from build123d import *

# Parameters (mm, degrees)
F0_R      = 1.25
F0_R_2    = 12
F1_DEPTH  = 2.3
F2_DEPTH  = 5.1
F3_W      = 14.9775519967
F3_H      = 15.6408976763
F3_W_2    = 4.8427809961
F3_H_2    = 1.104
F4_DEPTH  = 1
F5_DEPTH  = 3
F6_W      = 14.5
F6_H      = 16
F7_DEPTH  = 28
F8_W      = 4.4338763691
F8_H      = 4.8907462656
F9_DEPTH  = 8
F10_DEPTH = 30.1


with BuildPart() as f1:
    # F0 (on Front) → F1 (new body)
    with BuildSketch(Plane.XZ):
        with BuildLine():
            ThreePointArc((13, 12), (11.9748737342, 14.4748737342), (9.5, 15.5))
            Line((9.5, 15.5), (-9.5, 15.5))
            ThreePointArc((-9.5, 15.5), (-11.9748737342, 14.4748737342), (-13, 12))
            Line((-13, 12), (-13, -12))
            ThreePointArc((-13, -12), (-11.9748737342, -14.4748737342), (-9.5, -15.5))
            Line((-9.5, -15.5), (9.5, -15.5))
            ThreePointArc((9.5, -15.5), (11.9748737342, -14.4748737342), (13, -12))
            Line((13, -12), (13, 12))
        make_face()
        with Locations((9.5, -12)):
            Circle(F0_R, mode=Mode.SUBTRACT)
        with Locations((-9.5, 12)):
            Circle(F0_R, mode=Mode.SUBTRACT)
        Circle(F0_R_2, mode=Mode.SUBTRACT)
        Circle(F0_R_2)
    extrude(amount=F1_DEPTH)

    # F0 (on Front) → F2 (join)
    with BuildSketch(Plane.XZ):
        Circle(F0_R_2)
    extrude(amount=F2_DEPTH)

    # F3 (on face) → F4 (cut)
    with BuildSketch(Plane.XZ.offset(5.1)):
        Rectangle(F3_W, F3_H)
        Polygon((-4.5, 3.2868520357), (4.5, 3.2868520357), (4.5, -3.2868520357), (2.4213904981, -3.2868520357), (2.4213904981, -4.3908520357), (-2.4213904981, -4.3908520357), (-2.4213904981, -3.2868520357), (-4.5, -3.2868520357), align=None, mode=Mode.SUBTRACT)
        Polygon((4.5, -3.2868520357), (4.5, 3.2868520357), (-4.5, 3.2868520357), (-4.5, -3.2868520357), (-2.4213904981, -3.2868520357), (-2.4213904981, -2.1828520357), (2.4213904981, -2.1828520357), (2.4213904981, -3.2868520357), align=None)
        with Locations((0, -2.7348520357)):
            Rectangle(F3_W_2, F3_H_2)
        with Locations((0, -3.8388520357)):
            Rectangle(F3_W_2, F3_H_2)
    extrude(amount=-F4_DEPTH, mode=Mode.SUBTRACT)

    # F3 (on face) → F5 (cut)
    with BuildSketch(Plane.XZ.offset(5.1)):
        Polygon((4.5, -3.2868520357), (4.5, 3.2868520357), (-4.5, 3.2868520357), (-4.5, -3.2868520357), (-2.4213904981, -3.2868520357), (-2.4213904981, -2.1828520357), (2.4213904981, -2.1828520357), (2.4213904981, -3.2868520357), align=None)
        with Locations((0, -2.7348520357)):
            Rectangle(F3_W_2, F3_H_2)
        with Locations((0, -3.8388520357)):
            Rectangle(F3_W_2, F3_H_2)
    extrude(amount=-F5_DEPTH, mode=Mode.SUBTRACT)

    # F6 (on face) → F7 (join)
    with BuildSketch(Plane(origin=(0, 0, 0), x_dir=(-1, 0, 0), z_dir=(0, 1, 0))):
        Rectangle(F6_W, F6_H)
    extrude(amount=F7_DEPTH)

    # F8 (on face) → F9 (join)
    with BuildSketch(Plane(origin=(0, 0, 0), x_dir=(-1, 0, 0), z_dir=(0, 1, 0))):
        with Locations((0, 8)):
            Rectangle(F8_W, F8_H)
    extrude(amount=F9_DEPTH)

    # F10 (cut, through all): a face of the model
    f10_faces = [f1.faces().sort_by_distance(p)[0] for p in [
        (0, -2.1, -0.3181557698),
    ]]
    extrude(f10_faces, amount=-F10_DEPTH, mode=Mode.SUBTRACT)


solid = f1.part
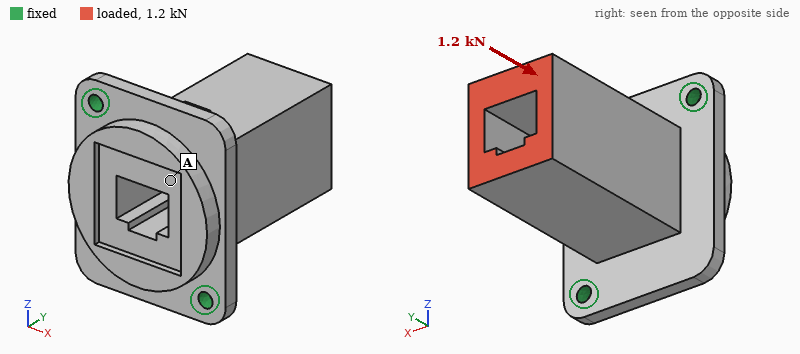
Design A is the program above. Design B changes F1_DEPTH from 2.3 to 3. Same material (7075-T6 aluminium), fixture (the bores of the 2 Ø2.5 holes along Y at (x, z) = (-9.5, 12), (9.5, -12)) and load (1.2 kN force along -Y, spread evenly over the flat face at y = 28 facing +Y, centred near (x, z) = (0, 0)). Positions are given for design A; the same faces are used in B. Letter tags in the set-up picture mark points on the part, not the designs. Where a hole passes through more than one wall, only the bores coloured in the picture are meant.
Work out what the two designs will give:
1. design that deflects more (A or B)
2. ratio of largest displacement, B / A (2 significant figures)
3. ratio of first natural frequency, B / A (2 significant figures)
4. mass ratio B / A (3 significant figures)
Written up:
A
0.78
1.3
1.03
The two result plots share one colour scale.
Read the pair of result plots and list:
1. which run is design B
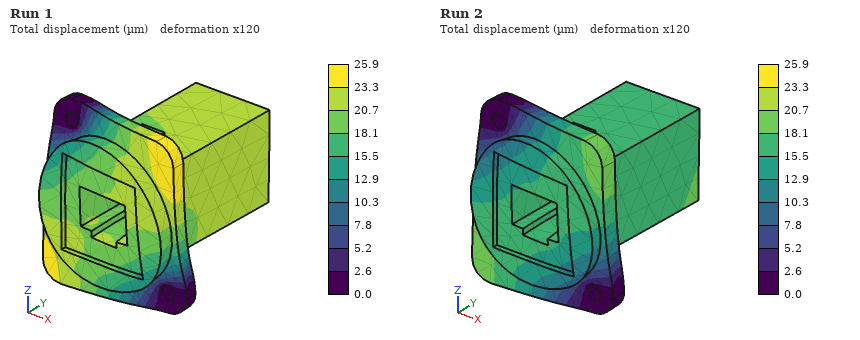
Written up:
Run 2
